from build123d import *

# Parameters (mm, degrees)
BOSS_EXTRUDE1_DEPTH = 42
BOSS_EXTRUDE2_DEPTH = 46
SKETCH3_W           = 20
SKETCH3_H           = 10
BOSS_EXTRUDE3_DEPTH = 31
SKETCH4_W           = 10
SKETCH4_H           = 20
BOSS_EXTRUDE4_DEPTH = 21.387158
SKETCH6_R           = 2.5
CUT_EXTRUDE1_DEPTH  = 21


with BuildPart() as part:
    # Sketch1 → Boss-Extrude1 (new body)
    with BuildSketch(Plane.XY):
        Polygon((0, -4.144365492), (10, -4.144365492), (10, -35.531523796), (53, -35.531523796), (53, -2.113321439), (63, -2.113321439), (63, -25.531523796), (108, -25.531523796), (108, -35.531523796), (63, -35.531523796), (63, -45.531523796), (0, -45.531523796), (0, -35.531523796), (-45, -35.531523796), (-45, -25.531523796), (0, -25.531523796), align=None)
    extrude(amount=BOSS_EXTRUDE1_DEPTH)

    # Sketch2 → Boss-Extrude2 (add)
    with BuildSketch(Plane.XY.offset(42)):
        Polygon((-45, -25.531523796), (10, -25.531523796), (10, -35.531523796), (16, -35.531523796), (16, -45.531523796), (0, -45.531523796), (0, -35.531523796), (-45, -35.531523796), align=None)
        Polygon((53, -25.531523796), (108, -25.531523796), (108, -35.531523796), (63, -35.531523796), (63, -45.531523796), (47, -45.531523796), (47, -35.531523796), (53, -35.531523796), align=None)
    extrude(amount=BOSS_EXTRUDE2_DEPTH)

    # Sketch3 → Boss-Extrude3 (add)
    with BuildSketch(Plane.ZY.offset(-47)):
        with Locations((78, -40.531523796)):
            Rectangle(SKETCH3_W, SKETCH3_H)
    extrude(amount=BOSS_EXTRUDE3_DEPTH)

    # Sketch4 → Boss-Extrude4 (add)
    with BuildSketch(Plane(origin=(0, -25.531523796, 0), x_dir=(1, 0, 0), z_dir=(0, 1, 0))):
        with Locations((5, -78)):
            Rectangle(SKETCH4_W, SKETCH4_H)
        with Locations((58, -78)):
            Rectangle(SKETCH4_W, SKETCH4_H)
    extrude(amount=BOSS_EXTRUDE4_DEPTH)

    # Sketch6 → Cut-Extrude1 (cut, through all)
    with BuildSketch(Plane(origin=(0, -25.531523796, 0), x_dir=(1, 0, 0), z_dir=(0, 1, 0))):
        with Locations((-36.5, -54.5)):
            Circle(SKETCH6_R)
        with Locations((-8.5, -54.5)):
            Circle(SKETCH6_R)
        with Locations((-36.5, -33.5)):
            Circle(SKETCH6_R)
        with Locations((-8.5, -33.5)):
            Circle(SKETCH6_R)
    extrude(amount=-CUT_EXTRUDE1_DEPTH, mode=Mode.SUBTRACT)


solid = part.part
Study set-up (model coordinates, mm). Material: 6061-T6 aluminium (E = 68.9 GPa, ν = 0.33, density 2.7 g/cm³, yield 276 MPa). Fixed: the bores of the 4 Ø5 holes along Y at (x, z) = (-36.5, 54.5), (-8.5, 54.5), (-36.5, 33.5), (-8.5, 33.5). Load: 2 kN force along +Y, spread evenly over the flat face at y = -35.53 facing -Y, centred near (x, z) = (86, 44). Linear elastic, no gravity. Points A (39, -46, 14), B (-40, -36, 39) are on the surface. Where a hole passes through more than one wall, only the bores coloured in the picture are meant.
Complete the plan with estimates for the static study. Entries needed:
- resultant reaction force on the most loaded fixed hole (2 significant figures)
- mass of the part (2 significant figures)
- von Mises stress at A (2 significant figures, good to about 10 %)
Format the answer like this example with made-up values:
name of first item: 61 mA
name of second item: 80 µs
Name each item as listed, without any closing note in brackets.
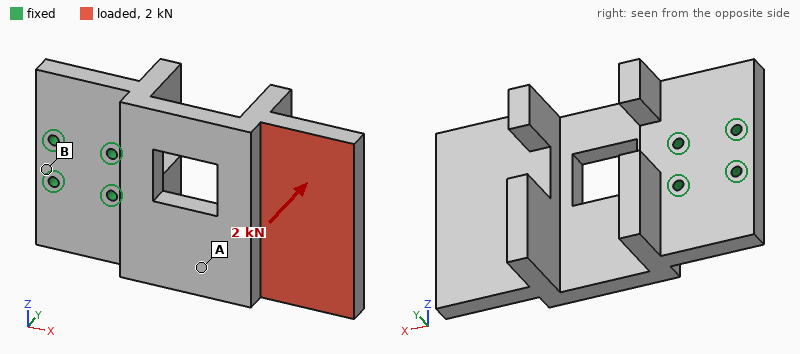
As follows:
resultant reaction force on the most loaded fixed hole: 2.6 kN
mass of the part: 460 g
von Mises stress at A: 79 MPa
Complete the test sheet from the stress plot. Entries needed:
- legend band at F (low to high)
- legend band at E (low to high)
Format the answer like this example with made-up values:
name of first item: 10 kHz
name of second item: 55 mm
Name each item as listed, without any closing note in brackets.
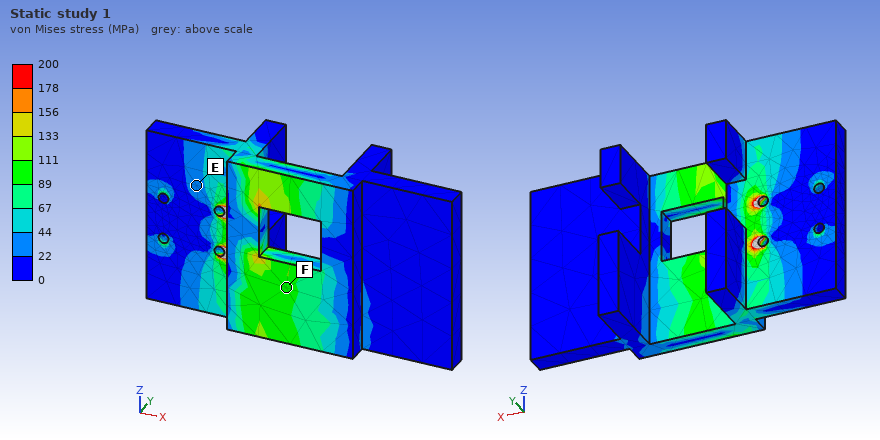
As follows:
legend band at F: 89 to 111 MPa
legend band at E: 22 to 44 MPa
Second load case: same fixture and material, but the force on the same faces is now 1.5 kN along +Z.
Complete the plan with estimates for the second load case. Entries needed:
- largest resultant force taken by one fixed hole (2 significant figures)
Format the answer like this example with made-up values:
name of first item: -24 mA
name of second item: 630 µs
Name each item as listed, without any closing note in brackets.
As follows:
largest resultant force taken by one fixed hole: 2.8 kN
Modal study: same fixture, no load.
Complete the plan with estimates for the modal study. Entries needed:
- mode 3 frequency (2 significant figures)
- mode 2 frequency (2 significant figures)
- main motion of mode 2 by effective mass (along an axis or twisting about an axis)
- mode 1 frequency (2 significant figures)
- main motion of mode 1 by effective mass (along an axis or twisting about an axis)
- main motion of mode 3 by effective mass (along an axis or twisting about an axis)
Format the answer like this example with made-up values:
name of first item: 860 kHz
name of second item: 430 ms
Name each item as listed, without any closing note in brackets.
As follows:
mode 3 frequency: 2000 Hz
mode 2 frequency: 1200 Hz
main motion of mode 2 by effective mass: along Z
mode 1 frequency: 470 Hz
main motion of mode 1 by effective mass: along Y
main motion of mode 3 by effective mass: along Z
